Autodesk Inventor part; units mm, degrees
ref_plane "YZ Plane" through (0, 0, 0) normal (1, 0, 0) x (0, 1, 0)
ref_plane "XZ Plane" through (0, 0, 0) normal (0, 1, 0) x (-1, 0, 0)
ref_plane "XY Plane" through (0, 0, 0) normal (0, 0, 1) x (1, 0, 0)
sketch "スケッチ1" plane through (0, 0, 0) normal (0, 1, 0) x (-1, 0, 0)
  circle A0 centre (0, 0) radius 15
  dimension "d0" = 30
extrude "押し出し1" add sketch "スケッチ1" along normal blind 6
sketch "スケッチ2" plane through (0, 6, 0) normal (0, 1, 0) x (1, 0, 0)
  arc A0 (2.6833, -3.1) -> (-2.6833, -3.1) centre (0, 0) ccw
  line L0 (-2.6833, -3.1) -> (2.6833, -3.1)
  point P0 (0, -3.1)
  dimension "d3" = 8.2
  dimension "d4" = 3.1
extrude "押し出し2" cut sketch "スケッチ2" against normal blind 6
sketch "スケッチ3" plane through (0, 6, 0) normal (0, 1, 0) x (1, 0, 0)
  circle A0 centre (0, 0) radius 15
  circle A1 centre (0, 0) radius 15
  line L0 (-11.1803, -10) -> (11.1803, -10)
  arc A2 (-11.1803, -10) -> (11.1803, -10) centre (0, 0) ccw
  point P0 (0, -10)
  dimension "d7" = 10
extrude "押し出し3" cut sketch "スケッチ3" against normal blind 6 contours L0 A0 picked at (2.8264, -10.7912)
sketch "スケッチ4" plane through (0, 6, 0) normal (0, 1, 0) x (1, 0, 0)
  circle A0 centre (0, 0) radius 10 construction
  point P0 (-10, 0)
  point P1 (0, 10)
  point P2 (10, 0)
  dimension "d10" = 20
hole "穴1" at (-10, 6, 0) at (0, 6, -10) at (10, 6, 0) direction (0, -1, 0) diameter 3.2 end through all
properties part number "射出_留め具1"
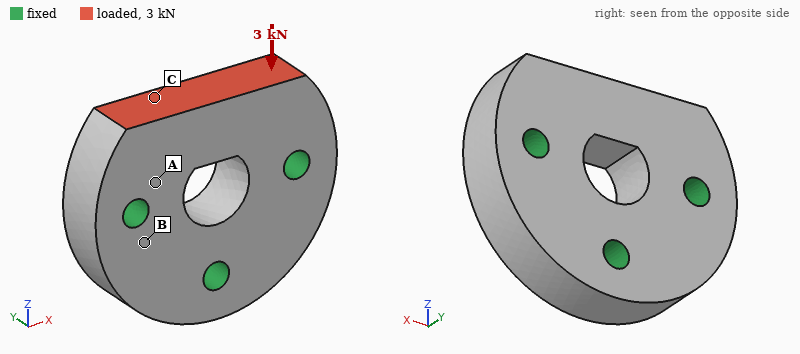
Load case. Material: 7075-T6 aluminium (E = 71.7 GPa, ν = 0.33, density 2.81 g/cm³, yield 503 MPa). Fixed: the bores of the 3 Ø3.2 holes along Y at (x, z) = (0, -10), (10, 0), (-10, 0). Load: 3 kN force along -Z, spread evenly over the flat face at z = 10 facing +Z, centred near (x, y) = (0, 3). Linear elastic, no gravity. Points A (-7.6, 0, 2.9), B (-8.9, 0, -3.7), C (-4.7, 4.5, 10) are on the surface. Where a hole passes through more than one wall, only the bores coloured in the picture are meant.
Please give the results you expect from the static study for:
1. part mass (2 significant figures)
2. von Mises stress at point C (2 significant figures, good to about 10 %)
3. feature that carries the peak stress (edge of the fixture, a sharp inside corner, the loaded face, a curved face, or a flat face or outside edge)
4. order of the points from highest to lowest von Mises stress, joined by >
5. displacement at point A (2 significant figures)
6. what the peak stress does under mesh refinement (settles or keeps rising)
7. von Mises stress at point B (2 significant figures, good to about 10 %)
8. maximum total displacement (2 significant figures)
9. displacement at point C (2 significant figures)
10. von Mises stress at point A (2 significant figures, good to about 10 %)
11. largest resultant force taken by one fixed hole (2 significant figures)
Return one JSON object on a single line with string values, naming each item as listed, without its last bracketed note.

{"part mass": "9.4 g", "von Mises stress at point C": "20 MPa", "feature that carries the peak stress": "edge of the fixture", "order of the points from highest to lowest von Mises stress, joined by >": "A > C > B", "displacement at point A": "1.5 µm", "what the peak stress does under mesh refinement": "keeps rising", "von Mises stress at point B": "9.8 MPa", "maximum total displacement": "6.3 µm", "displacement at point C": "5.2 µm", "von Mises stress at point A": "33 MPa", "largest resultant force taken by one fixed hole": "1.4 kN"}
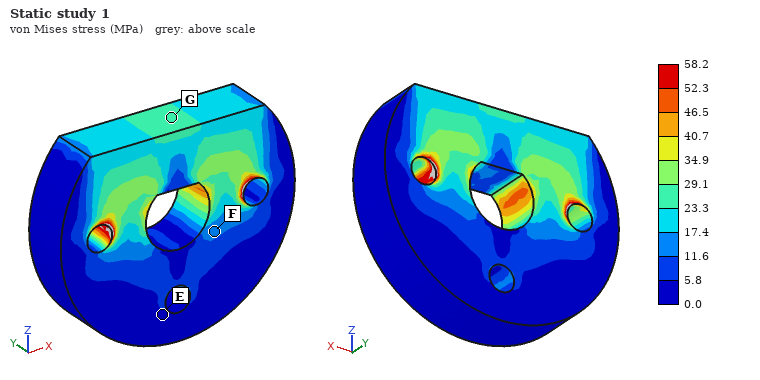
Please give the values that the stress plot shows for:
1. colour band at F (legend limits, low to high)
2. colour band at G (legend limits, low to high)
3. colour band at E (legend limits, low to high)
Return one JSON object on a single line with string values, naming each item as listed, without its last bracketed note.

{"colour band at F": "11.6 to 17.4 MPa", "colour band at G": "23.3 to 29.1 MPa", "colour band at E": "0.0 to 5.8 MPa"}
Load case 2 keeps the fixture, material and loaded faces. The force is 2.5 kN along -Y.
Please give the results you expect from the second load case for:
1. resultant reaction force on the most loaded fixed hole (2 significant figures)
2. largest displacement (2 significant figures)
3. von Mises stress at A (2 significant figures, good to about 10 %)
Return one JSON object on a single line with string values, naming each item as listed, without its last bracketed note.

{"resultant reaction force on the most loaded fixed hole": "1.4 kN", "largest displacement": "54 µm", "von Mises stress at A": "150 MPa"}
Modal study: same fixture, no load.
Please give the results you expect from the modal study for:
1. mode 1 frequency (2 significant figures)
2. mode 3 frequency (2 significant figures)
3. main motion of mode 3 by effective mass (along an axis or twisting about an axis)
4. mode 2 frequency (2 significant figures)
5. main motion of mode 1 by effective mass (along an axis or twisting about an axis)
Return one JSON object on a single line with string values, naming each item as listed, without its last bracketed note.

{"mode 1 frequency": "34 kHz", "mode 3 frequency": "60 kHz", "main motion of mode 3 by effective mass": "along X", "mode 2 frequency": "53 kHz", "main motion of mode 1 by effective mass": "along Y"}
